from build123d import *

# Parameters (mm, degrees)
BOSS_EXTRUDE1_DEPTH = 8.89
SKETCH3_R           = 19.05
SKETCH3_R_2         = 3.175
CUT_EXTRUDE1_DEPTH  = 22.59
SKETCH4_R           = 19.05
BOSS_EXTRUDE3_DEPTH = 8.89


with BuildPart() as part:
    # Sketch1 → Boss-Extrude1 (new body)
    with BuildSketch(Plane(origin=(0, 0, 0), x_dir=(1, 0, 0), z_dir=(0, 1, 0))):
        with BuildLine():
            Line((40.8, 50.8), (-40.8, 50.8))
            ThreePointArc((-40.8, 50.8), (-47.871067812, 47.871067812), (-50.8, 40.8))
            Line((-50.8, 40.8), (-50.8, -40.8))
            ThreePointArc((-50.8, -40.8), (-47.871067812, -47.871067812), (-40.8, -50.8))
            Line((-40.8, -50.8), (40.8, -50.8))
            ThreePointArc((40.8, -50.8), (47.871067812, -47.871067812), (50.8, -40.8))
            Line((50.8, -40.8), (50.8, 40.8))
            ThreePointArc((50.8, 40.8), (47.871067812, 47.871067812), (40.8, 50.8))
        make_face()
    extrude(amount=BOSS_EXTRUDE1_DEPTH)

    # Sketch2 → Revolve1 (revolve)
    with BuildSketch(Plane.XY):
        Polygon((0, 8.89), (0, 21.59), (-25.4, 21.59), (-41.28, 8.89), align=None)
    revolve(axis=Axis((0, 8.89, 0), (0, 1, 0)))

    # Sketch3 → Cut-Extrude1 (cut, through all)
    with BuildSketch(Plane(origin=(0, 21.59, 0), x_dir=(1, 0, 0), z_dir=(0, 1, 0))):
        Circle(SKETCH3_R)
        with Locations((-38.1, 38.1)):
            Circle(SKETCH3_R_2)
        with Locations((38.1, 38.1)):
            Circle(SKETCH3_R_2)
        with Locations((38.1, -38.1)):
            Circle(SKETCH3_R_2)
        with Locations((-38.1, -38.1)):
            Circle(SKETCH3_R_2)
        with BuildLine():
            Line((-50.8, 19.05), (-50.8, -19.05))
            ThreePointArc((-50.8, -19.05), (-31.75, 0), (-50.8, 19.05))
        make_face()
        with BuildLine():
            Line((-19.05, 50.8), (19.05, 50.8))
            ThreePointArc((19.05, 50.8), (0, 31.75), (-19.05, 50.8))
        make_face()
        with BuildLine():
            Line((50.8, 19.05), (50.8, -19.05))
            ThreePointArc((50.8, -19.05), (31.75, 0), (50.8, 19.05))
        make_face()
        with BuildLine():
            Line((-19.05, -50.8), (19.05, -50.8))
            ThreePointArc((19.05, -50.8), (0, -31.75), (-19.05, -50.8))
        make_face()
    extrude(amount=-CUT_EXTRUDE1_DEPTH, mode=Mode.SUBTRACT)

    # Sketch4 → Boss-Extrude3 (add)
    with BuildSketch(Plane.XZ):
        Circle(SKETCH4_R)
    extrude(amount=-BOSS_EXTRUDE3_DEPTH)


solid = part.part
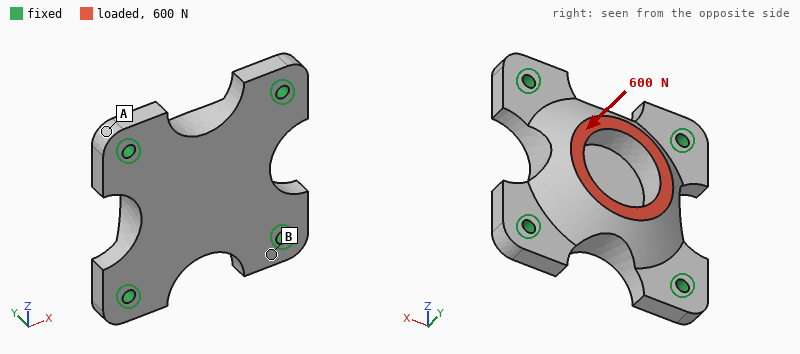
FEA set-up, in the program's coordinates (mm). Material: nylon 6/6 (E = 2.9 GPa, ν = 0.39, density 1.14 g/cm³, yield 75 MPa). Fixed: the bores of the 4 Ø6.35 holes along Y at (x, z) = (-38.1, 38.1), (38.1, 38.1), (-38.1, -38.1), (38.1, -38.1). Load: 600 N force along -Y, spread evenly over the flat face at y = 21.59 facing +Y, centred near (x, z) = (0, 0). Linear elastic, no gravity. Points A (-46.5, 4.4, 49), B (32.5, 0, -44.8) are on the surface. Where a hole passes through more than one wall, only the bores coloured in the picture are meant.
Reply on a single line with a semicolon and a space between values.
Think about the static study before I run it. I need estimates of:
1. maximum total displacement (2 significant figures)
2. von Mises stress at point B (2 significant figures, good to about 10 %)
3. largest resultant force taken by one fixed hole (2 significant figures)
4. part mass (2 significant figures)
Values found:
63 µm; 1.4 MPa; 180 N; 110 g
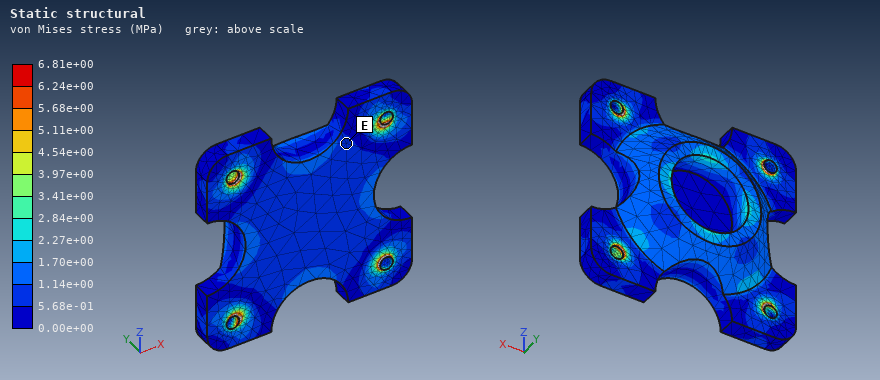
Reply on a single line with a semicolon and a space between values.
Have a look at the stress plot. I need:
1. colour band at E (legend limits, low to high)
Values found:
5.68e-01 to 1.14e+00 MPa
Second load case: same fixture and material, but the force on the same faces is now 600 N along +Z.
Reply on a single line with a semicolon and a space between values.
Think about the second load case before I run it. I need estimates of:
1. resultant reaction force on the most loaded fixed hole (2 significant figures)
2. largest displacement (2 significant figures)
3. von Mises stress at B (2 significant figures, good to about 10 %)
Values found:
190 N; 31 µm; 0.90 MPa
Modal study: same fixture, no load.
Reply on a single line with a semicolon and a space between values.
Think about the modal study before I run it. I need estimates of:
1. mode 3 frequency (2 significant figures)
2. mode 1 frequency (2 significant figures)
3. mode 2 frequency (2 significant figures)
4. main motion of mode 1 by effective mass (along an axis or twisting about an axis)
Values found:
3300 Hz; 2000 Hz; 3300 Hz; along Y
